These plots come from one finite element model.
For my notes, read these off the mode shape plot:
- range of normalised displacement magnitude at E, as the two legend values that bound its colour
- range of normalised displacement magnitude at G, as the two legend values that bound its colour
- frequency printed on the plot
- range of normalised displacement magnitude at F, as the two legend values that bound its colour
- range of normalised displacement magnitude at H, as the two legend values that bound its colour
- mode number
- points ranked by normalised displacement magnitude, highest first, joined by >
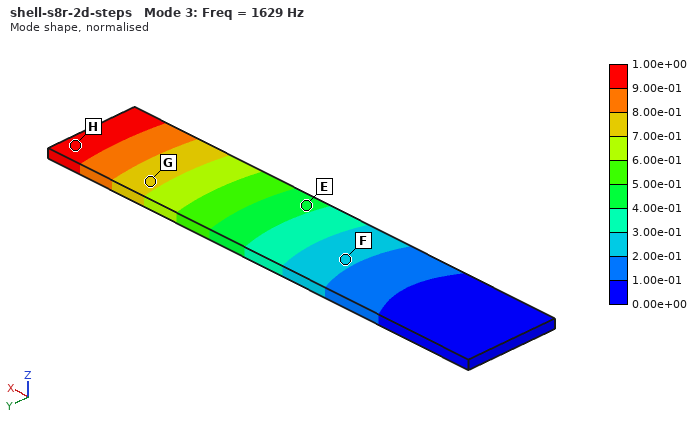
4.00e-01 to 5.00e-01
7.00e-01 to 8.00e-01
1629 Hz
2.00e-01 to 3.00e-01
9.00e-01 to 1.00e+00
3
H > G > E > F
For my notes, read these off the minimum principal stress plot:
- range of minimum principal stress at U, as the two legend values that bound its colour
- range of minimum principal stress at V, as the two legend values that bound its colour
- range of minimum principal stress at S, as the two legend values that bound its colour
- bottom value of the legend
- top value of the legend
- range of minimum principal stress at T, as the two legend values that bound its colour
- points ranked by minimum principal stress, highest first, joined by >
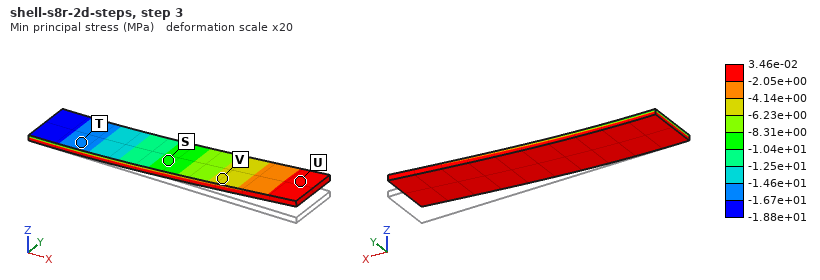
-2.05e+00 to 3.46e-02 MPa
-6.23e+00 to -4.14e+00 MPa
-1.04e+01 to -8.31e+00 MPa
-1.88e+01 MPa
3.46e-02 MPa
-1.67e+01 to -1.46e+01 MPa
U > V > S > T
